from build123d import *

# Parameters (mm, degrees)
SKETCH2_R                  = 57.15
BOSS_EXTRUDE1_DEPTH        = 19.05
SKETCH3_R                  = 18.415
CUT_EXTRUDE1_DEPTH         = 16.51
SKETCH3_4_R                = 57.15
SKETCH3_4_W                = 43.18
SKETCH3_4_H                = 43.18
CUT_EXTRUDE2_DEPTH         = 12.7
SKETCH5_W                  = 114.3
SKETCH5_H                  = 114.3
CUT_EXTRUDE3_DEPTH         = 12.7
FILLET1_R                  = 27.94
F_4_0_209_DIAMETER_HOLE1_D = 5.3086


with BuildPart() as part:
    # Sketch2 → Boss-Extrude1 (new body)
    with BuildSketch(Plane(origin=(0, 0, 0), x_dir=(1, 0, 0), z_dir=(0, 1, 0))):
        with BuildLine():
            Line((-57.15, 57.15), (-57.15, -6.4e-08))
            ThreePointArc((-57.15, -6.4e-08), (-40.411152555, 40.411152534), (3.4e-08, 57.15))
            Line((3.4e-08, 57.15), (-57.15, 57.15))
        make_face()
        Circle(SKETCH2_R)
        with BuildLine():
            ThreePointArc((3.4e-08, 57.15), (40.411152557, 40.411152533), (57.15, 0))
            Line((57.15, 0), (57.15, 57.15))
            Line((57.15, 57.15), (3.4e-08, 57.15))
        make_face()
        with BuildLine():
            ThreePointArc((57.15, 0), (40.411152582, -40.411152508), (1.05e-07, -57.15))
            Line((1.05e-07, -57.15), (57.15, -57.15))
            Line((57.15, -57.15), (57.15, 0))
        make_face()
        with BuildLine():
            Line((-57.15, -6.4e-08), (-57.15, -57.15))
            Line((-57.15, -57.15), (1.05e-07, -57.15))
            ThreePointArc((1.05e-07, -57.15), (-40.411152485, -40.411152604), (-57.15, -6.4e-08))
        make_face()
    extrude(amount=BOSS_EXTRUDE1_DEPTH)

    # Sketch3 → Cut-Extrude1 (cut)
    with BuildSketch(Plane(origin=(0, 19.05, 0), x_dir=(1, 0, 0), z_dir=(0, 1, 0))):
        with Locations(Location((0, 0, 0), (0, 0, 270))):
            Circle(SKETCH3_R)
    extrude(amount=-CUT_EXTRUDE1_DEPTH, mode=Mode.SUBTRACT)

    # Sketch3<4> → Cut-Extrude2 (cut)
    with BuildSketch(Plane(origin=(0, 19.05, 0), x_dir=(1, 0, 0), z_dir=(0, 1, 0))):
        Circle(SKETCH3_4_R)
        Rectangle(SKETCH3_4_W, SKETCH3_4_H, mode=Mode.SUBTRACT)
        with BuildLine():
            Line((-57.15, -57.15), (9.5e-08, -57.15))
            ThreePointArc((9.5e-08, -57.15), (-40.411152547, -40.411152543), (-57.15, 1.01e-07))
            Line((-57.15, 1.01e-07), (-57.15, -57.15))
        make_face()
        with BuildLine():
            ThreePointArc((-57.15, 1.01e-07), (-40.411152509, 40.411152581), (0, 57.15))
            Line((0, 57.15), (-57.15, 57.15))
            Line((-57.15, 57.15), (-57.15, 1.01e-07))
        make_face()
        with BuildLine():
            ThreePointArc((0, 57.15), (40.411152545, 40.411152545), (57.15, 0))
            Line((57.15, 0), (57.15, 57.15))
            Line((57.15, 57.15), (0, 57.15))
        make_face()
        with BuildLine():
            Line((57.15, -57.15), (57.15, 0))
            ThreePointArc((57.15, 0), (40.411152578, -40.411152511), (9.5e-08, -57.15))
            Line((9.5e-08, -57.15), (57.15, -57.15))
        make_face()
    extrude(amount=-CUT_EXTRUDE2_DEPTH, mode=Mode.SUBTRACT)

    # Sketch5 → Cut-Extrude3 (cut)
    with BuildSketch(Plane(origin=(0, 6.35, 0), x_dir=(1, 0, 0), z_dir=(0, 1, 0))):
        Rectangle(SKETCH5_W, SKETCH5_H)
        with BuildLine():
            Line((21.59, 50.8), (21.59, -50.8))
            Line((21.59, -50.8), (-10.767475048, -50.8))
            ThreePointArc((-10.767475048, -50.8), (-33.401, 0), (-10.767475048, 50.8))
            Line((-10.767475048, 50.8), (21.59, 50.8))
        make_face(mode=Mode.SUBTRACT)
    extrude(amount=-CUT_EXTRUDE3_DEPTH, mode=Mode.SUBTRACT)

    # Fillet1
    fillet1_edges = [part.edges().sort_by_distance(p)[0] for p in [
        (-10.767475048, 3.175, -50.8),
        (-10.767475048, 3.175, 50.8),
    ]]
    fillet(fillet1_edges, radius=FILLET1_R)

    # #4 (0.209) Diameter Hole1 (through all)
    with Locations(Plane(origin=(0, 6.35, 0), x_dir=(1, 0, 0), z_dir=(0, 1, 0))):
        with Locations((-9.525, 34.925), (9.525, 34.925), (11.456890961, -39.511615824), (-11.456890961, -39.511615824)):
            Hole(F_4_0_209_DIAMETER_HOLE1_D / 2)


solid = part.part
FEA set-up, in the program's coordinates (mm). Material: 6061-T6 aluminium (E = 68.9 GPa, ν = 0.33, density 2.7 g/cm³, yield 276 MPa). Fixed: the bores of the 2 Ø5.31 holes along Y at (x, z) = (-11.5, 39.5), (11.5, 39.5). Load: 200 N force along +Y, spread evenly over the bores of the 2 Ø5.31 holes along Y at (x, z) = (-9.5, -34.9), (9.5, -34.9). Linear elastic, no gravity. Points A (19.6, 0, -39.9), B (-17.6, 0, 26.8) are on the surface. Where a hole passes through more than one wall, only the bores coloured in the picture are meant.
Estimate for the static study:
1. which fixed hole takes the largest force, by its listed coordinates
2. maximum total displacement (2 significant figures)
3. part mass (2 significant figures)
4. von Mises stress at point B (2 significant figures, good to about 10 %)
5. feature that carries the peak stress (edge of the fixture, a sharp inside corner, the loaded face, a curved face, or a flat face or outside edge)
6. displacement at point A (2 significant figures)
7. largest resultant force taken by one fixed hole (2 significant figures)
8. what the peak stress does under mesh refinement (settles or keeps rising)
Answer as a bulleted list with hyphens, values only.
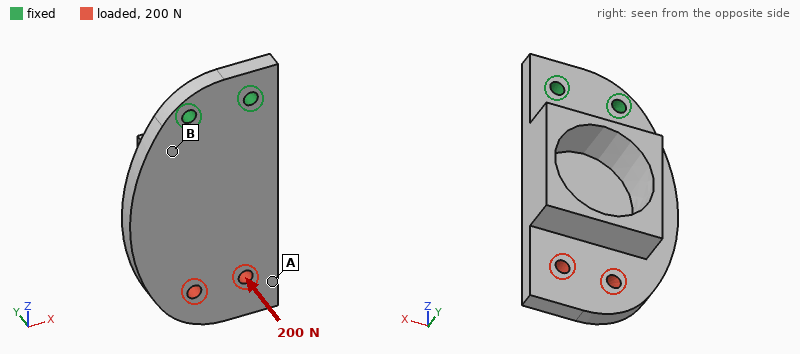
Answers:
- (-11.5, 39.5)
- 0.36 mm
- 98 g
- 33 MPa
- edge of the fixture
- 0.30 mm
- 110 N
- keeps rising
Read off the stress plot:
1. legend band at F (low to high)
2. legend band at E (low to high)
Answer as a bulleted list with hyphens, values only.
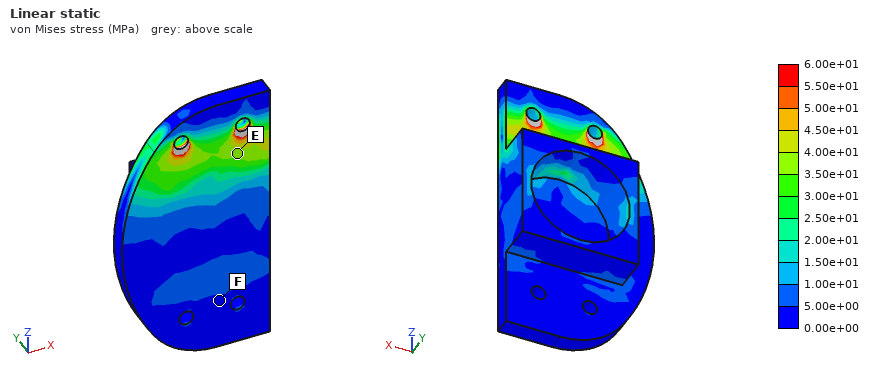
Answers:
- 0.00e+00 to 5.00e+00 MPa
- 3.50e+01 to 4.00e+01 MPa
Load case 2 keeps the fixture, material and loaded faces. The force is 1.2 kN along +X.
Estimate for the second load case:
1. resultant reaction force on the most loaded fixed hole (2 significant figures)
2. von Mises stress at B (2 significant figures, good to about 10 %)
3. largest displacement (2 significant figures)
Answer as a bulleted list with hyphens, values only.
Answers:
- 3.5 kN
- 20 MPa
- 100 µm
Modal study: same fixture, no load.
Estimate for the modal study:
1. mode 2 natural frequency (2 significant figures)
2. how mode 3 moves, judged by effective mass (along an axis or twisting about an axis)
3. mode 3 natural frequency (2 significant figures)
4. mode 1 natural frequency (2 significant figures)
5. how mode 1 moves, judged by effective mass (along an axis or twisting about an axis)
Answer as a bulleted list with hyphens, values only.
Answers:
- 2400 Hz
- along X
- 3200 Hz
- 720 Hz
- along Y
